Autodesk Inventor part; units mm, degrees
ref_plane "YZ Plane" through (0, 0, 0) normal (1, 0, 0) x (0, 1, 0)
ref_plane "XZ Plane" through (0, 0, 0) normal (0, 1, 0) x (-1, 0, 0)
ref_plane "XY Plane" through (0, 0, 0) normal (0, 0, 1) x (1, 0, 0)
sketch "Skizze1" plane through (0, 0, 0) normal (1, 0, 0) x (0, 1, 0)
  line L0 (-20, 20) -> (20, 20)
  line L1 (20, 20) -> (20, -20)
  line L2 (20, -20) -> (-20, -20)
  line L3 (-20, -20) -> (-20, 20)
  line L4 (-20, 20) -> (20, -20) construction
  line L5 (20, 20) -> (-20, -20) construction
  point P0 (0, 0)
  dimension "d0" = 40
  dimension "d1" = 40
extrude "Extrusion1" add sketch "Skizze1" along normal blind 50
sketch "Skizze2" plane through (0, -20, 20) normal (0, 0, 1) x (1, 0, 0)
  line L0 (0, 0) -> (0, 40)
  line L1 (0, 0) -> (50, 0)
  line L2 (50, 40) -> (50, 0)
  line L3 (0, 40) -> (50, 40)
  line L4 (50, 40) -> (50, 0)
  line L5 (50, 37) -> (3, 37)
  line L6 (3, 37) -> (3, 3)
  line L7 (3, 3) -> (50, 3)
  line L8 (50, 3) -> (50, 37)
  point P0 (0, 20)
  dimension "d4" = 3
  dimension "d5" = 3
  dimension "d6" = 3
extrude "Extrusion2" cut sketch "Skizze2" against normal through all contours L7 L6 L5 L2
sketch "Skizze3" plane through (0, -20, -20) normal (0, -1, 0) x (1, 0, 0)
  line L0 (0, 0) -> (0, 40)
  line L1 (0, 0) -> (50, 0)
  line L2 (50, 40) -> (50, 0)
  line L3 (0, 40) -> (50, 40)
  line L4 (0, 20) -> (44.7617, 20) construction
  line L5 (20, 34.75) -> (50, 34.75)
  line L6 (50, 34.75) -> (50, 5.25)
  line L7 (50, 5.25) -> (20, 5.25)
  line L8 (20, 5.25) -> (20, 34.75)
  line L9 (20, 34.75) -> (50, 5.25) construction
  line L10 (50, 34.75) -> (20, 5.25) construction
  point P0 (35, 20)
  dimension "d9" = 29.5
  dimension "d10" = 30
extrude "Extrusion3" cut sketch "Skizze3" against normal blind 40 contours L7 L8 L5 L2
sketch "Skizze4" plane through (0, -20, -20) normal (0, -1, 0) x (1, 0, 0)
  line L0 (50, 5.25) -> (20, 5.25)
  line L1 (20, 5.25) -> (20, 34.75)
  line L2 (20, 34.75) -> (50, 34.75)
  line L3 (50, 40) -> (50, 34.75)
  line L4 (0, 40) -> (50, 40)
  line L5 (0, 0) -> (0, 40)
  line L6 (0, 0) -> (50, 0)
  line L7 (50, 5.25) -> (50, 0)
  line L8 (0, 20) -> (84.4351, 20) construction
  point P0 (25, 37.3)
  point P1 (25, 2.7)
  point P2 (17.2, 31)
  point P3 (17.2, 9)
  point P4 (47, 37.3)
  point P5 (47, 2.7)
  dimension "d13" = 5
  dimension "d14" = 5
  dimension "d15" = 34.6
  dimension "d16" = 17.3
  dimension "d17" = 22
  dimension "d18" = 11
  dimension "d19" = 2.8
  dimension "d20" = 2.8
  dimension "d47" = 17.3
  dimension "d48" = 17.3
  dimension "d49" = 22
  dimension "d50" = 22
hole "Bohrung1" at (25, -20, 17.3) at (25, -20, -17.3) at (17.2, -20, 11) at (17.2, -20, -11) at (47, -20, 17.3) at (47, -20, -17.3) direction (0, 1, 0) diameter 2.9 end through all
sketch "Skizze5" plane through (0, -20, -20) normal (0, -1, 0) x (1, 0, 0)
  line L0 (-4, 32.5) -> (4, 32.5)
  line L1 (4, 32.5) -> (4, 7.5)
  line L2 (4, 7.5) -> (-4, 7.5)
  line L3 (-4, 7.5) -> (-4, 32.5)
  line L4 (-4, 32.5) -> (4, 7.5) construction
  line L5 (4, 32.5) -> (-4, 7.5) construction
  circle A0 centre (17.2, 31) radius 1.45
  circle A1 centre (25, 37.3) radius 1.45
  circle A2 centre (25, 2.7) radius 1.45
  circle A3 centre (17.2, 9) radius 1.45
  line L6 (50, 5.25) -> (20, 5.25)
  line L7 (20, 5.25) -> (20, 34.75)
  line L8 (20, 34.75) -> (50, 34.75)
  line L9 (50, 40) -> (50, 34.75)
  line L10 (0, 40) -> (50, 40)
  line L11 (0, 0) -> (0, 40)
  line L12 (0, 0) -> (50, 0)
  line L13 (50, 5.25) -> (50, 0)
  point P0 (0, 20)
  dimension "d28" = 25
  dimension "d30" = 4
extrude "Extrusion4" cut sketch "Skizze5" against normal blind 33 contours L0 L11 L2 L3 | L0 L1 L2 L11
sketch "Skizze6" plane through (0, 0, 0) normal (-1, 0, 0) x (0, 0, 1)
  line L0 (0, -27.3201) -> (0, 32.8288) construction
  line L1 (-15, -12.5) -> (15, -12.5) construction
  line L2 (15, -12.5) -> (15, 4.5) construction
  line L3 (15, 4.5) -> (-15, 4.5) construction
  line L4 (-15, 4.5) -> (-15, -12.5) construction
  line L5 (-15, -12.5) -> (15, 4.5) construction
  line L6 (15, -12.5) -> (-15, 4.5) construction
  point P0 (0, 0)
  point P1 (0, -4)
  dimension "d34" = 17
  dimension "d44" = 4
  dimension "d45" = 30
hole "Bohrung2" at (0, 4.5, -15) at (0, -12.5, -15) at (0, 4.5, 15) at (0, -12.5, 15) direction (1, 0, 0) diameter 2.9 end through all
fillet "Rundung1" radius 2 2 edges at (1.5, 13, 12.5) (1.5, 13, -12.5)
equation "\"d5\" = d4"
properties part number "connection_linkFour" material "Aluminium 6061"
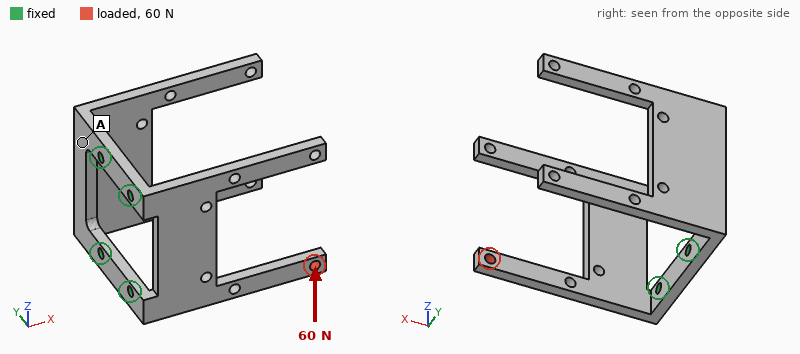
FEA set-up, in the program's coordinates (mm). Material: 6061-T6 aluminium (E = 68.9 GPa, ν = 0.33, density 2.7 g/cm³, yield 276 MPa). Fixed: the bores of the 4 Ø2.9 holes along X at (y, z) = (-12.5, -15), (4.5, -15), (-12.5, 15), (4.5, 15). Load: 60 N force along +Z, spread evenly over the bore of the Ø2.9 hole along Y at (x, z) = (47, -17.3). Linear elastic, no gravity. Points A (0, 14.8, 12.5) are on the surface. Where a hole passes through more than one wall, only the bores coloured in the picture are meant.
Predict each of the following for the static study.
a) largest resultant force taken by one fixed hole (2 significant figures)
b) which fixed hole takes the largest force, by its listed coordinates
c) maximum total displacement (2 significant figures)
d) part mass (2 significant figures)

110 N
(-12.5, 15)
0.29 mm
21 g
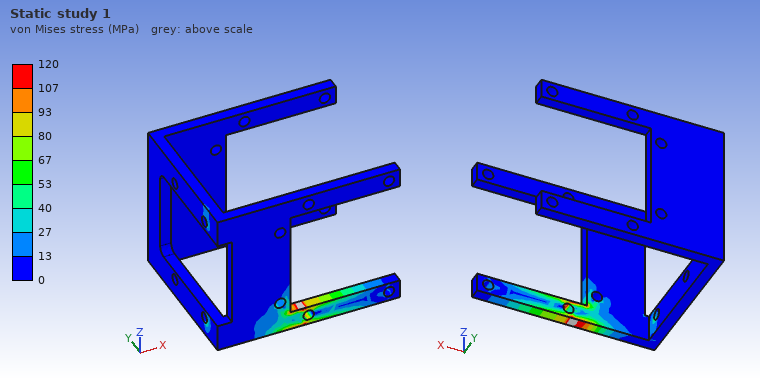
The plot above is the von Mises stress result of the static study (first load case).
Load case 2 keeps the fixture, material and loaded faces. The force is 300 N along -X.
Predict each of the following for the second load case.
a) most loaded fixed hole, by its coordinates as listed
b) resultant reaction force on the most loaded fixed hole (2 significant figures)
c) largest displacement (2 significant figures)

(-12.5, -15)
320 N
0.13 mm
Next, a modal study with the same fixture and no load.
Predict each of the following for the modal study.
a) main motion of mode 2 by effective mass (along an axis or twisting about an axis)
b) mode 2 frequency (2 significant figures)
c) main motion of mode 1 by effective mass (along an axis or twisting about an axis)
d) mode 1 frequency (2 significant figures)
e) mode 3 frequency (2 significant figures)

along Y
1100 Hz
along Y
950 Hz
1500 Hz
